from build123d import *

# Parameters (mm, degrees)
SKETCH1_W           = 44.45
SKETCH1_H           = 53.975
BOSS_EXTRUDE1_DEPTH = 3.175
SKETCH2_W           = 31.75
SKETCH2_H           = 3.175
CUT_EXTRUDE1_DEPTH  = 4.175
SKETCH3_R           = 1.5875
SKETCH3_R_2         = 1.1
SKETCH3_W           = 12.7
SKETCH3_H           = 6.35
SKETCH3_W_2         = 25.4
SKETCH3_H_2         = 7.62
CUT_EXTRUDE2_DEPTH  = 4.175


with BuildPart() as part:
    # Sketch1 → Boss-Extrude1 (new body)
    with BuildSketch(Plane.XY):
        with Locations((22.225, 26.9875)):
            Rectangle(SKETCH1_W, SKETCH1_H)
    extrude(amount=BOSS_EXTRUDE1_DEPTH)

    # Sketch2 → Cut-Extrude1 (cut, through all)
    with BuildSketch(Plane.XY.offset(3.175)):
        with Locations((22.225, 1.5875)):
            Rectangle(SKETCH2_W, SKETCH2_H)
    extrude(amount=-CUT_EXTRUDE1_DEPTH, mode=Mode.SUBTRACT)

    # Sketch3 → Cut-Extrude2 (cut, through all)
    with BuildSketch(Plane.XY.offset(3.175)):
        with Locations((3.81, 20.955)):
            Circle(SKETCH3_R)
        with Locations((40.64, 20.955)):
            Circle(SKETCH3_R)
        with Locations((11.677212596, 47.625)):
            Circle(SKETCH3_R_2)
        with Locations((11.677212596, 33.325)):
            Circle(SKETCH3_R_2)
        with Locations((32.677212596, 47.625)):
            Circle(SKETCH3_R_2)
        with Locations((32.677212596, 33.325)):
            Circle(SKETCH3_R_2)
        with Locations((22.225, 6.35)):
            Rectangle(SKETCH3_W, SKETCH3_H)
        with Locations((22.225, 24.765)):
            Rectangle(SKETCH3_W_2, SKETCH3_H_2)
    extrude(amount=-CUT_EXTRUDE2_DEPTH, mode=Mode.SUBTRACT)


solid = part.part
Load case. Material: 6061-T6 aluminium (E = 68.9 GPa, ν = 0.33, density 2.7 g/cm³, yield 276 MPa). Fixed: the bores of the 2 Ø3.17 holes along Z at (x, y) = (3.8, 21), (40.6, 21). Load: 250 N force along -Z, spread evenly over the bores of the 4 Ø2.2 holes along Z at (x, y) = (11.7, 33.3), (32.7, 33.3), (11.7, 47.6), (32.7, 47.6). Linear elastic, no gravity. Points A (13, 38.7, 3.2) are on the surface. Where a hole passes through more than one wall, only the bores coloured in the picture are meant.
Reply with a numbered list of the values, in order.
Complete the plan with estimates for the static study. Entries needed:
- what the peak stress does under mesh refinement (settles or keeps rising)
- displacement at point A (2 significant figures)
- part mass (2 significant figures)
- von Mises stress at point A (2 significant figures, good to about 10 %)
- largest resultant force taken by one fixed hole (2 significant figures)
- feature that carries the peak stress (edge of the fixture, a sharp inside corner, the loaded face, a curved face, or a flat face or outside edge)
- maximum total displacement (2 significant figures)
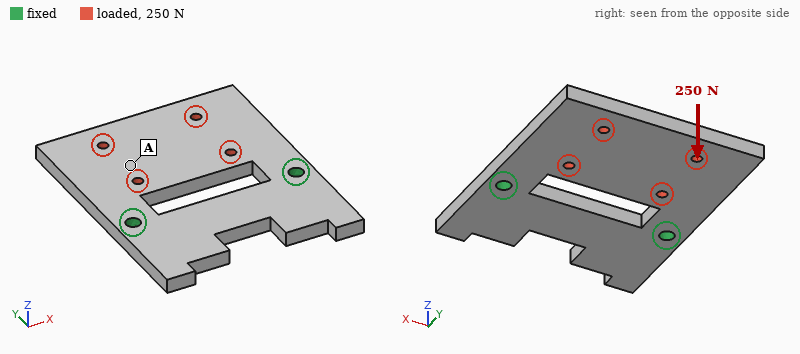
1. keeps rising
2. 0.15 mm
3. 17 g
4. 21 MPa
5. 130 N
6. edge of the fixture
7. 0.35 mm
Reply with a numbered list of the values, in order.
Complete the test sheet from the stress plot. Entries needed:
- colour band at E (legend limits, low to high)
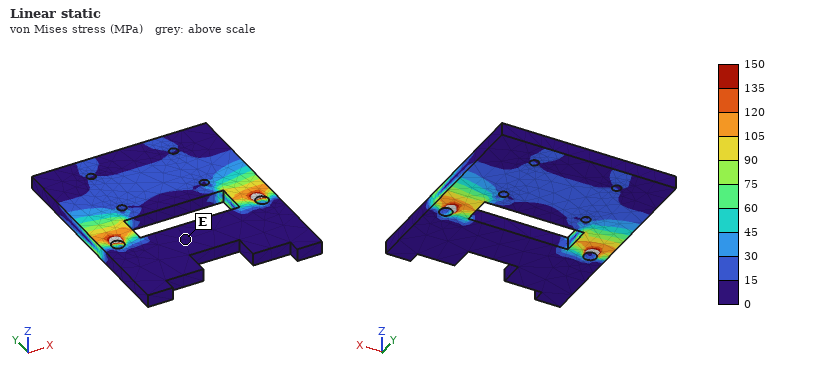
1. 0 to 15 MPa
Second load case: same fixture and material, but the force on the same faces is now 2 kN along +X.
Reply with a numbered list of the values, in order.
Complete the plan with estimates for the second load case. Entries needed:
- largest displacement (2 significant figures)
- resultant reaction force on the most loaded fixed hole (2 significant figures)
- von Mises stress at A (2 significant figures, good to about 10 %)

1. 40 µm
2. 1.3 kN
3. 25 MPa
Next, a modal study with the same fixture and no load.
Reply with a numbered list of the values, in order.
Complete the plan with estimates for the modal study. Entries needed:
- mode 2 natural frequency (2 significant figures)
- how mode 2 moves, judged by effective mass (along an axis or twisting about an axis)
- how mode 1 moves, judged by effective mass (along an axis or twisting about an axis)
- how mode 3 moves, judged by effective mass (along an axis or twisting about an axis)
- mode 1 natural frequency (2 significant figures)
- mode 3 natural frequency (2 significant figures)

1. 4500 Hz
2. twisting about Y
3. along Z
4. along Z
5. 1700 Hz
6. 5800 Hz
